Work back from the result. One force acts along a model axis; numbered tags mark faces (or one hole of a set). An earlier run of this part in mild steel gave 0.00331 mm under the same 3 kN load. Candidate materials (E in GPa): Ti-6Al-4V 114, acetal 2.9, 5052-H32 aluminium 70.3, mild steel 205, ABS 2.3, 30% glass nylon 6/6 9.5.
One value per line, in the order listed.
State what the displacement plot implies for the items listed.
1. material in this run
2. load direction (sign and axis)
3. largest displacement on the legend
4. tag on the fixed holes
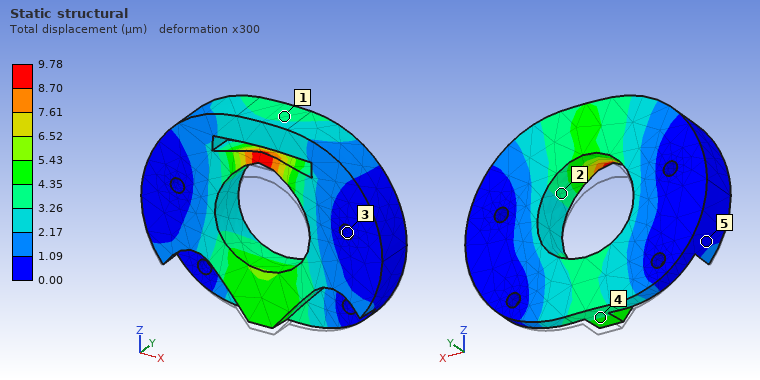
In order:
5052-H32 aluminium
+Z
9.78 µm
3
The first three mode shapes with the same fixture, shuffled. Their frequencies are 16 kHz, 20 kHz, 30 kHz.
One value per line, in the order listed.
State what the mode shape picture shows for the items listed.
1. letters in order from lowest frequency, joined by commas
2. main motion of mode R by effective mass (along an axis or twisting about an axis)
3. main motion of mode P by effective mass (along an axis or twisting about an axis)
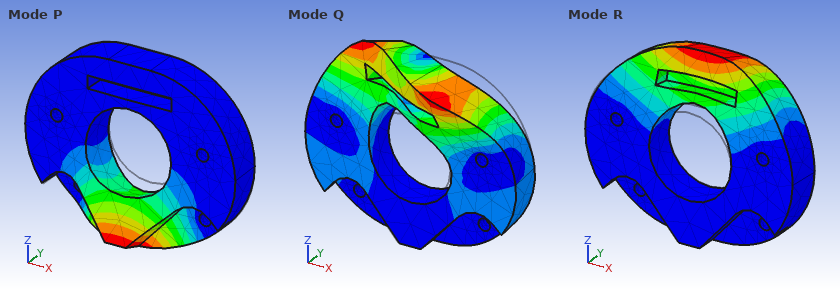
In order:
R, P, Q
along Y
along Y
